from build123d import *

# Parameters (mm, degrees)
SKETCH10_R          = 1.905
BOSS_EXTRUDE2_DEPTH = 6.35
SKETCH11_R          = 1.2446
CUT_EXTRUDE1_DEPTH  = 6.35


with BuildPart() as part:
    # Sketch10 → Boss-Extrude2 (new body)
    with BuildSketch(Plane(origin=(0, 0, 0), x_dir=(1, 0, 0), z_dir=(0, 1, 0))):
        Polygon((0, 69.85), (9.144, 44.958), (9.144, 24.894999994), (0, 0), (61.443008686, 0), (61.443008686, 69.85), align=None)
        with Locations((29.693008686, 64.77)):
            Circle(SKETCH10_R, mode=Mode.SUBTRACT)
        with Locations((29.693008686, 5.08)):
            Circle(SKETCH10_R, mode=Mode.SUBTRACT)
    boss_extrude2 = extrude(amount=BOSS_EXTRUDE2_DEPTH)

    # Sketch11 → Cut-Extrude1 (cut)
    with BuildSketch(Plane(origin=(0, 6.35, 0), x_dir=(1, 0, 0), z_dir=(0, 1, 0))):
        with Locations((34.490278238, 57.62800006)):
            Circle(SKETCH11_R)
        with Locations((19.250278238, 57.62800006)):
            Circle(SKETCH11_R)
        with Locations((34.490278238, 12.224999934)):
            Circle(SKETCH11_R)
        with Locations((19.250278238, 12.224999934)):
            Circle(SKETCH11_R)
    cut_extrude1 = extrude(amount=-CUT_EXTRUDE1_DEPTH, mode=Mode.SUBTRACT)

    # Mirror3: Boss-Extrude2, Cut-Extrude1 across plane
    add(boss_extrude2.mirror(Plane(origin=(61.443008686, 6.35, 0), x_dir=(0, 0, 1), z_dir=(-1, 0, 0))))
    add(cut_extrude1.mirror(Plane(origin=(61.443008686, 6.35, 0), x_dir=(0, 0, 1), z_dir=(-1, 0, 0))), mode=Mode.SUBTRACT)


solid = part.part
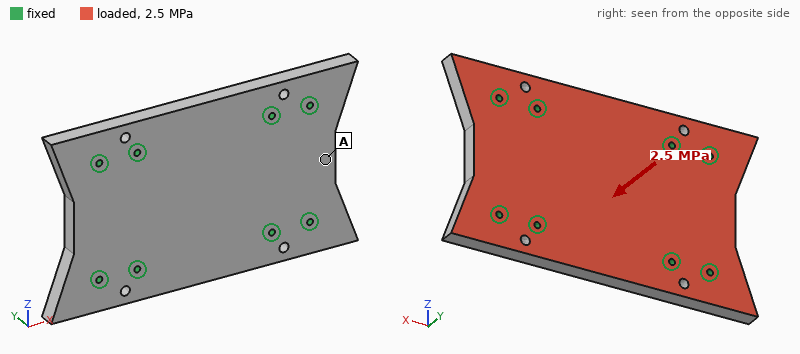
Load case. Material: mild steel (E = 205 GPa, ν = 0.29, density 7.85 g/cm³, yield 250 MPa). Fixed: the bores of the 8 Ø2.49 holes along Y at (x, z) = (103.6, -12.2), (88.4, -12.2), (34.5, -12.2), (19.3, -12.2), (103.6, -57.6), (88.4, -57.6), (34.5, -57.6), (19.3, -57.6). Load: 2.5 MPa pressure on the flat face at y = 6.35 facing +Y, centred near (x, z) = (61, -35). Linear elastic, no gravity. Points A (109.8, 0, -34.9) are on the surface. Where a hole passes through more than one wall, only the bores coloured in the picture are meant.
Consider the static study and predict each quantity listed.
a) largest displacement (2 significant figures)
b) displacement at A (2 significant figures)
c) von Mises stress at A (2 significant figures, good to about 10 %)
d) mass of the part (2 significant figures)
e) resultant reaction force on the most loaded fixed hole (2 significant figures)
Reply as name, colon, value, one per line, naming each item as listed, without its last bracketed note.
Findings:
largest displacement: 28 µm
displacement at A: 9.3 µm
von Mises stress at A: 31 MPa
mass of the part: 380 g
resultant reaction force on the most loaded fixed hole: 3.2 kN
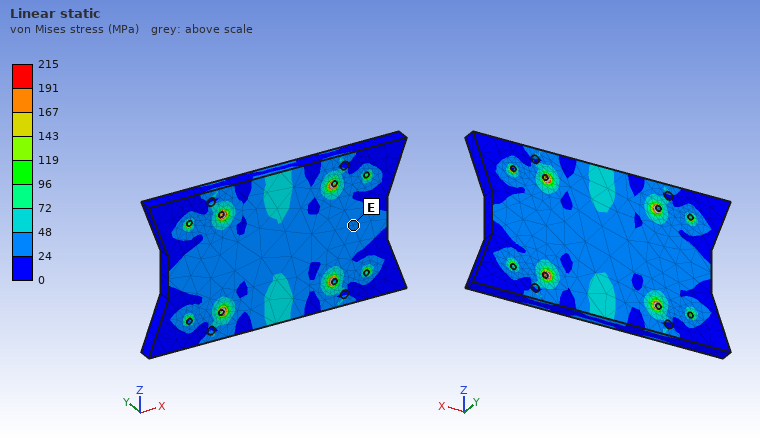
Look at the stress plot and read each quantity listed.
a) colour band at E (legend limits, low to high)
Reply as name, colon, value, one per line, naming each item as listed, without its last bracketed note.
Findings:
colour band at E: 24 to 48 MPa
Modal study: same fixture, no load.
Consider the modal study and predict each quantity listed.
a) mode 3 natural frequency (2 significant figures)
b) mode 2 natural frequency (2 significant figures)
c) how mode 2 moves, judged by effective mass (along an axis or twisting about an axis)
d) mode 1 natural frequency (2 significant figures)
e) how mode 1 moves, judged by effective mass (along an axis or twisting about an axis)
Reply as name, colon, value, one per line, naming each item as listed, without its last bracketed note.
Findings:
mode 3 natural frequency: 11 kHz
mode 2 natural frequency: 10000 Hz
how mode 2 moves, judged by effective mass: twisting about X
mode 1 natural frequency: 7900 Hz
how mode 1 moves, judged by effective mass: along Y
